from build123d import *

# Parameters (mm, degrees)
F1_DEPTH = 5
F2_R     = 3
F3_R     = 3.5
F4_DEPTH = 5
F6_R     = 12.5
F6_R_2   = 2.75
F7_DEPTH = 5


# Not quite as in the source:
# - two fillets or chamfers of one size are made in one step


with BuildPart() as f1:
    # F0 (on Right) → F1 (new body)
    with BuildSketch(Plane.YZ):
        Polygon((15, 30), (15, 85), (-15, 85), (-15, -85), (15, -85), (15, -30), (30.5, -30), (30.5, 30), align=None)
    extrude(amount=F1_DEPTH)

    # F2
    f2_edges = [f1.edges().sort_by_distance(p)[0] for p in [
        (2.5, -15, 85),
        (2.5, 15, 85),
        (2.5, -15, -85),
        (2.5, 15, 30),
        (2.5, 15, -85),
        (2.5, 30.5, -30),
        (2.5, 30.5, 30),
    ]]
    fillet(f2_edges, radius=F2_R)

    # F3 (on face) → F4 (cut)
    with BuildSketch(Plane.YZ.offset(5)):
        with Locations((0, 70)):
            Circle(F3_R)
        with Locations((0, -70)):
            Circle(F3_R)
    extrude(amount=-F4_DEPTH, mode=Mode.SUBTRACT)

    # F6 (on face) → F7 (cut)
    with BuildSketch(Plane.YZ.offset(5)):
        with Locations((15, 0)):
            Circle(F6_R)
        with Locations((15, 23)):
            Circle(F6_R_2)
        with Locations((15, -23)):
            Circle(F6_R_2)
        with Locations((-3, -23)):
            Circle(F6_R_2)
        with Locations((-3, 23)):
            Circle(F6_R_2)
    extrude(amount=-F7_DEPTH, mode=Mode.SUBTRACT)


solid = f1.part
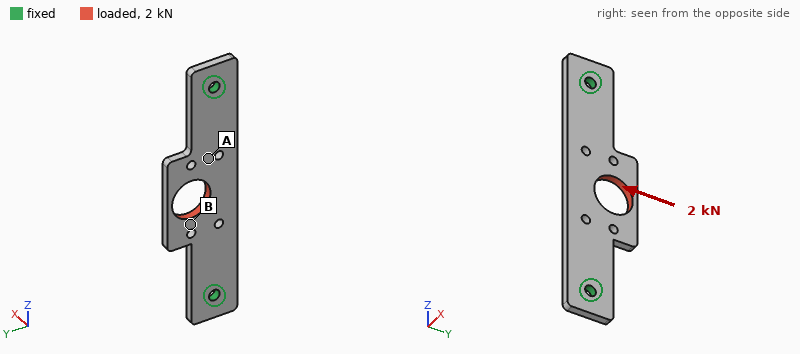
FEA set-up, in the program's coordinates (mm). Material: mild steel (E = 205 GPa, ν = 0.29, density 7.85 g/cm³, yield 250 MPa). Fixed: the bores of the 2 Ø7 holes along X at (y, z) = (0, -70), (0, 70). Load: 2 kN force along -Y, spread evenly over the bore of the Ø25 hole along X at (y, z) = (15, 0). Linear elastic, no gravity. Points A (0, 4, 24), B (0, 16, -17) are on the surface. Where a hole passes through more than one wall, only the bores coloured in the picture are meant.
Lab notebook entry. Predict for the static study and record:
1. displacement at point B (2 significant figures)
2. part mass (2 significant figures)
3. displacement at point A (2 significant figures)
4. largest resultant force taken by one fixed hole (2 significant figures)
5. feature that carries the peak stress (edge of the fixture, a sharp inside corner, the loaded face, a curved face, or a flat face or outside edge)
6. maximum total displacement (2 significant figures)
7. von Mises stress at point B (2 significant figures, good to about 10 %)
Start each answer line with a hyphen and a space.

- 21 µm
- 210 g
- 20 µm
- 1.0 kN
- edge of the fixture
- 24 µm
- 23 MPa
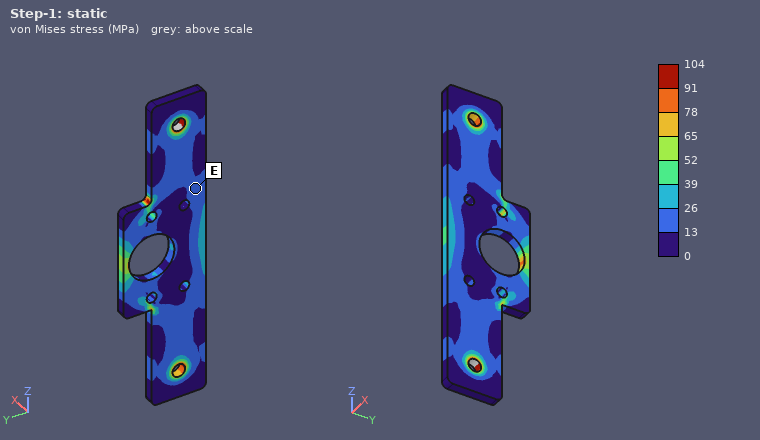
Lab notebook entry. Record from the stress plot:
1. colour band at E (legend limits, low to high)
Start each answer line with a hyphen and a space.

- 13 to 26 MPa
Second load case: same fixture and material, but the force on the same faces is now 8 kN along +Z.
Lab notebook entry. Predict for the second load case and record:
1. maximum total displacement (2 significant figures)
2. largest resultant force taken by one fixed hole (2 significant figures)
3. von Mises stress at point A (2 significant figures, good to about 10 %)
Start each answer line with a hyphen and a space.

- 25 µm
- 4.2 kN
- 23 MPa
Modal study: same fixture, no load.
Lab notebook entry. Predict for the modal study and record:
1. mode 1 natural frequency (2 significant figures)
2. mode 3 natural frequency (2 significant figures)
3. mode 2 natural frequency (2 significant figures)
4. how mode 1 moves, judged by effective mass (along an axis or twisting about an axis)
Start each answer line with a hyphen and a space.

- 1200 Hz
- 3300 Hz
- 2300 Hz
- along X
